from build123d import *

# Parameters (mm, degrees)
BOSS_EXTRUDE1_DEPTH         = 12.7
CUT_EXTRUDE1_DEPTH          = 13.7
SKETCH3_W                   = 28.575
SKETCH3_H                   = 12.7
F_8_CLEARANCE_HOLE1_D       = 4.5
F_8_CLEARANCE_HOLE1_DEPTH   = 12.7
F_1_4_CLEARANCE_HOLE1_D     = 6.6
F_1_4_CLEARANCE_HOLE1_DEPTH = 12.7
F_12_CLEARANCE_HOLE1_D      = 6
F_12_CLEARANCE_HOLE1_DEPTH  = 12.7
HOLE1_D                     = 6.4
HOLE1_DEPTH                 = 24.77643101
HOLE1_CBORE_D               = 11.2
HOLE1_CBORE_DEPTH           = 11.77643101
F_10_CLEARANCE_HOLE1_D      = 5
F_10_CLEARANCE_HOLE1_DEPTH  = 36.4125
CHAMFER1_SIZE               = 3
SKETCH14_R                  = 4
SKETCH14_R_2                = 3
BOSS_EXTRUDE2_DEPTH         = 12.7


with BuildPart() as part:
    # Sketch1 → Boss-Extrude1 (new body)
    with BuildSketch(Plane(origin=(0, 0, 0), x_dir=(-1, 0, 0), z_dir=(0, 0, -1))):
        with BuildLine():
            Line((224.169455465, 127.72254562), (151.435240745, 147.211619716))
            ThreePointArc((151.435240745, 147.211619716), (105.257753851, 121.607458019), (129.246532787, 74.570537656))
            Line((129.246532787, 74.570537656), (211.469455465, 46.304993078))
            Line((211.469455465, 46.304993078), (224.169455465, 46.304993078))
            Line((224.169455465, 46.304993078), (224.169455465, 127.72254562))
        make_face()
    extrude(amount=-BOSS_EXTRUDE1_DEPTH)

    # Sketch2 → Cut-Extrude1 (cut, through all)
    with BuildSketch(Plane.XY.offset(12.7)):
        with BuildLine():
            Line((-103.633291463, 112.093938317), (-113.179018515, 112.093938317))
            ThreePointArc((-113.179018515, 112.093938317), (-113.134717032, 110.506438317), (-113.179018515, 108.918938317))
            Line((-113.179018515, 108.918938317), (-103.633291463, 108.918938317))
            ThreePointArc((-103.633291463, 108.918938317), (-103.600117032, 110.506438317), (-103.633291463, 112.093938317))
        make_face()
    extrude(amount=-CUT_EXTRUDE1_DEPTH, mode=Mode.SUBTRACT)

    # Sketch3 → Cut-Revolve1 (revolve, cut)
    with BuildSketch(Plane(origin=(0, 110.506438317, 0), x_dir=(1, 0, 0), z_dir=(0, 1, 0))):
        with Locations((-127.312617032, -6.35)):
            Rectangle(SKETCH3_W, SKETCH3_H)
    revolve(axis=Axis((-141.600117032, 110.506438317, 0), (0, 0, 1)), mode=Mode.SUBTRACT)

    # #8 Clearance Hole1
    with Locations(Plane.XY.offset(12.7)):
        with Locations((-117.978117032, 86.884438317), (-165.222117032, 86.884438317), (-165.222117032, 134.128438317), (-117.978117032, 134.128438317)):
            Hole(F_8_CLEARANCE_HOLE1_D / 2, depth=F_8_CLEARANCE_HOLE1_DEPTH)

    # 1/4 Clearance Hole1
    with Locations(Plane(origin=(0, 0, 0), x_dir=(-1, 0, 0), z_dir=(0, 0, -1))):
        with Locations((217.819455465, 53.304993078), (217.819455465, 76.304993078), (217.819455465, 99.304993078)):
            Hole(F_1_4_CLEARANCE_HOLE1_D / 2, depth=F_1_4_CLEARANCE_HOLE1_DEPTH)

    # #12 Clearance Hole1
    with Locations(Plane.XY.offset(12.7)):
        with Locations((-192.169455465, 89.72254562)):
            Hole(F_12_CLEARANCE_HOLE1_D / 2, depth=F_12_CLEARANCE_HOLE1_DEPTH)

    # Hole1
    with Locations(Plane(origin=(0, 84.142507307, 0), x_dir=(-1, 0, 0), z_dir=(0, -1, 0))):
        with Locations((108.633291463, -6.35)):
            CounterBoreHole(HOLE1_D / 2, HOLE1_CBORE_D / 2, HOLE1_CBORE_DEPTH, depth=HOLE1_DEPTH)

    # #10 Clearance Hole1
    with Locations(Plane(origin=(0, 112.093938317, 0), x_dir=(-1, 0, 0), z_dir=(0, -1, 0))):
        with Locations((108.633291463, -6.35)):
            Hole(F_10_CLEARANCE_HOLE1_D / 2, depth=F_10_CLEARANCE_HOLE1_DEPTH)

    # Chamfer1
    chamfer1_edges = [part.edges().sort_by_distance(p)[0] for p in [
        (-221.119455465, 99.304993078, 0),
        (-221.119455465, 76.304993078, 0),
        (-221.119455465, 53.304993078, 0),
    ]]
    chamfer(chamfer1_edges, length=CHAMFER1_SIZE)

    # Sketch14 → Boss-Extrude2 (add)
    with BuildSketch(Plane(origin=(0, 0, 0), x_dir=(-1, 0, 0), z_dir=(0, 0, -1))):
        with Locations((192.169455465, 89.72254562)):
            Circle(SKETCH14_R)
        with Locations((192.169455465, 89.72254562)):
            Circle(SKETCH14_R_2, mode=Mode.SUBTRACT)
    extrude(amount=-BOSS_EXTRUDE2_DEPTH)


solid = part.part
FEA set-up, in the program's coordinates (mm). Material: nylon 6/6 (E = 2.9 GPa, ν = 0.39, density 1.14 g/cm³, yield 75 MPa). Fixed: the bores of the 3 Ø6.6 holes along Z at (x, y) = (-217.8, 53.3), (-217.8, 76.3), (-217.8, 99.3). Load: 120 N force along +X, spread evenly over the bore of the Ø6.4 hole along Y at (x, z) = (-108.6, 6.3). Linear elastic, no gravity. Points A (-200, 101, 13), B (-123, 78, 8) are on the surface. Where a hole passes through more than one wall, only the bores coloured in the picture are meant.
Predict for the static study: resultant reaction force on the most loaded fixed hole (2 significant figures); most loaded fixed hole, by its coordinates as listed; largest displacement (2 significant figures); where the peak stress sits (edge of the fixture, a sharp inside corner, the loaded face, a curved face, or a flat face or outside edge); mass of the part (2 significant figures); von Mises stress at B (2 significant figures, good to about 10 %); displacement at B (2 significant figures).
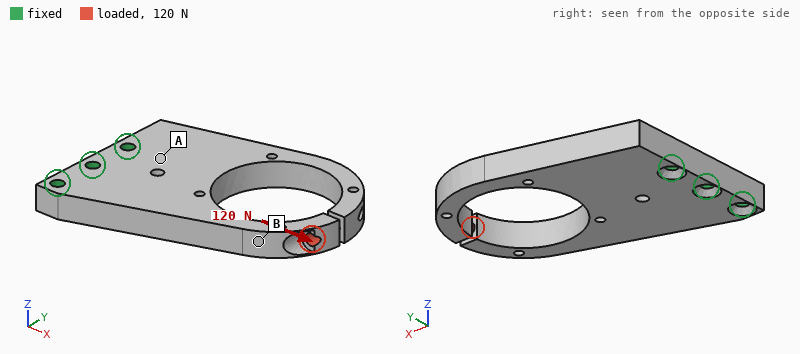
110 N
(-217.8, 99.3)
1.7 mm
a curved face
89 g
11 MPa
0.38 mm
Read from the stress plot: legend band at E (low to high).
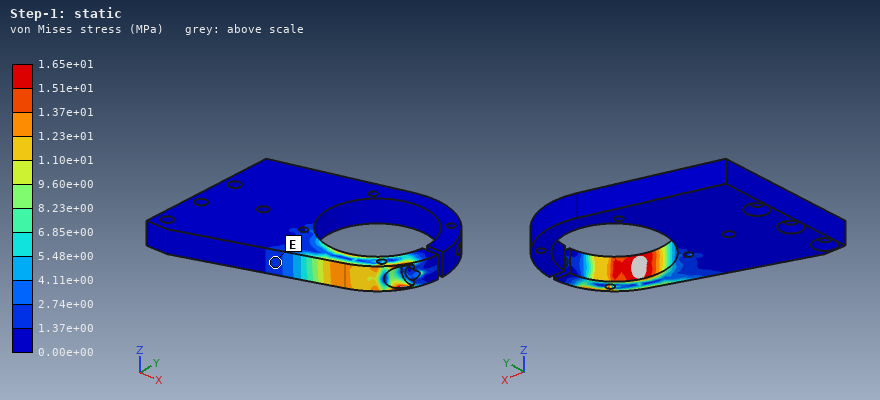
1.37e+00 to 2.74e+00 MPa
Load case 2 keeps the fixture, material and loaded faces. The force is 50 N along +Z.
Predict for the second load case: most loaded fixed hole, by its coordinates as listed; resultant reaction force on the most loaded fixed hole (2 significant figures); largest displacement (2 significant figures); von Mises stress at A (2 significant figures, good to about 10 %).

(-217.8, 76.3)
45 N
1.8 mm
2.1 MPa
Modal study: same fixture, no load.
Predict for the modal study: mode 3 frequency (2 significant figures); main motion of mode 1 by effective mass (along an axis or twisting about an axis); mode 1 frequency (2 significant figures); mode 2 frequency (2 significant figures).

500 Hz
along Z
320 Hz
480 Hz
